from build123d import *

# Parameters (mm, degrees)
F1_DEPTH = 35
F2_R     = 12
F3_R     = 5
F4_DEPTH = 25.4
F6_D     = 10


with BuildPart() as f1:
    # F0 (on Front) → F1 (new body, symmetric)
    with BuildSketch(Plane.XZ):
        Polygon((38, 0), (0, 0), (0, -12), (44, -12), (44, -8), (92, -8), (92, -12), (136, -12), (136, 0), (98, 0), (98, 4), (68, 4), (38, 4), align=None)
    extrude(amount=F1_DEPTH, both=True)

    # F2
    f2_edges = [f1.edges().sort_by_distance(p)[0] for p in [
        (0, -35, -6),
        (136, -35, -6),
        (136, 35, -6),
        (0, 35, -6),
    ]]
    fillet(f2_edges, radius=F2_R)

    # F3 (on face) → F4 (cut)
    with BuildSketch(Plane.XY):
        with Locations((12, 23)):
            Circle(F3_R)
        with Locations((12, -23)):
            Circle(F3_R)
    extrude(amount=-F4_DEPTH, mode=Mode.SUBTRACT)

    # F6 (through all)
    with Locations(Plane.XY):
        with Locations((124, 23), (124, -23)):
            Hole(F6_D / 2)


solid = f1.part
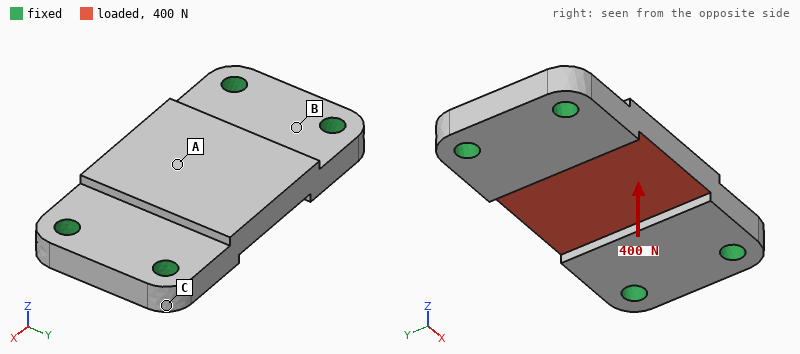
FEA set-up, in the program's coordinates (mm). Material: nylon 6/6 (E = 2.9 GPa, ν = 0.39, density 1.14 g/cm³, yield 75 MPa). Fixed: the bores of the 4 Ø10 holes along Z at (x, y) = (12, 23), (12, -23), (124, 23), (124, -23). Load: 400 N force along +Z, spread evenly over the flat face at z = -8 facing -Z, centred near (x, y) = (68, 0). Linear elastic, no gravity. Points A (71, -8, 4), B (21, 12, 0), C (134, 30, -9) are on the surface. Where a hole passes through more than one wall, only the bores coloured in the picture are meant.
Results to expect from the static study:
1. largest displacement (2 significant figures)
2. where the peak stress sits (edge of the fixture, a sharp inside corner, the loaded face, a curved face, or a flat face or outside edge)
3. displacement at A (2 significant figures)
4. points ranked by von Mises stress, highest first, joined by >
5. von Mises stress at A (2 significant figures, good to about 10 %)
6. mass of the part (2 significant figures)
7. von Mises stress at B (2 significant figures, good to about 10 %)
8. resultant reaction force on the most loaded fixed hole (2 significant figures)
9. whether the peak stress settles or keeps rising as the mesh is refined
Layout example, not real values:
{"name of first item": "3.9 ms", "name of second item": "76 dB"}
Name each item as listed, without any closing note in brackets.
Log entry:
{"largest displacement": "81 µm", "where the peak stress sits": "edge of the fixture", "displacement at A": "71 µm", "points ranked by von Mises stress, highest first, joined by >": "A > B > C", "von Mises stress at A": "1.8 MPa", "mass of the part": "130 g", "von Mises stress at B": "0.96 MPa", "resultant reaction force on the most loaded fixed hole": "170 N", "whether the peak stress settles or keeps rising as the mesh is refined": "keeps rising"}
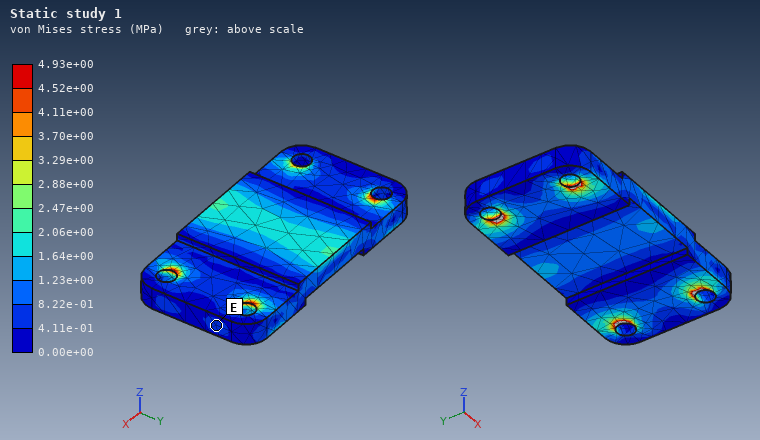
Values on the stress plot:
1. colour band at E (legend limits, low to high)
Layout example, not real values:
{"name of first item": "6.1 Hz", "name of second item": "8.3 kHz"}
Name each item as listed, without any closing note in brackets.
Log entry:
{"colour band at E": "4.11e-01 to 8.22e-01 MPa"}
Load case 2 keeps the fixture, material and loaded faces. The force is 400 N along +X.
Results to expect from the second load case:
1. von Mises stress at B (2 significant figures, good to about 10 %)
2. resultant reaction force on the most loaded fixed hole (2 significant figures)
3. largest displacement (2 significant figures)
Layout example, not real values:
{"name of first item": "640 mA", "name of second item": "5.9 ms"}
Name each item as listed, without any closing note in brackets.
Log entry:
{"von Mises stress at B": "0.31 MPa", "resultant reaction force on the most loaded fixed hole": "100 N", "largest displacement": "6.2 µm"}
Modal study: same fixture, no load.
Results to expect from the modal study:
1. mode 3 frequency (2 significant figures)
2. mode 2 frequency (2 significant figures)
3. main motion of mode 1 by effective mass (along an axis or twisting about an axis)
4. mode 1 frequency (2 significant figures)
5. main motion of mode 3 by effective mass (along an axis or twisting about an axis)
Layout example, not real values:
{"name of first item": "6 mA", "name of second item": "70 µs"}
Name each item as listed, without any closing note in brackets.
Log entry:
{"mode 3 frequency": "3600 Hz", "mode 2 frequency": "2200 Hz", "main motion of mode 1 by effective mass": "along Z", "mode 1 frequency": "1600 Hz", "main motion of mode 3 by effective mass": "along Y"}
